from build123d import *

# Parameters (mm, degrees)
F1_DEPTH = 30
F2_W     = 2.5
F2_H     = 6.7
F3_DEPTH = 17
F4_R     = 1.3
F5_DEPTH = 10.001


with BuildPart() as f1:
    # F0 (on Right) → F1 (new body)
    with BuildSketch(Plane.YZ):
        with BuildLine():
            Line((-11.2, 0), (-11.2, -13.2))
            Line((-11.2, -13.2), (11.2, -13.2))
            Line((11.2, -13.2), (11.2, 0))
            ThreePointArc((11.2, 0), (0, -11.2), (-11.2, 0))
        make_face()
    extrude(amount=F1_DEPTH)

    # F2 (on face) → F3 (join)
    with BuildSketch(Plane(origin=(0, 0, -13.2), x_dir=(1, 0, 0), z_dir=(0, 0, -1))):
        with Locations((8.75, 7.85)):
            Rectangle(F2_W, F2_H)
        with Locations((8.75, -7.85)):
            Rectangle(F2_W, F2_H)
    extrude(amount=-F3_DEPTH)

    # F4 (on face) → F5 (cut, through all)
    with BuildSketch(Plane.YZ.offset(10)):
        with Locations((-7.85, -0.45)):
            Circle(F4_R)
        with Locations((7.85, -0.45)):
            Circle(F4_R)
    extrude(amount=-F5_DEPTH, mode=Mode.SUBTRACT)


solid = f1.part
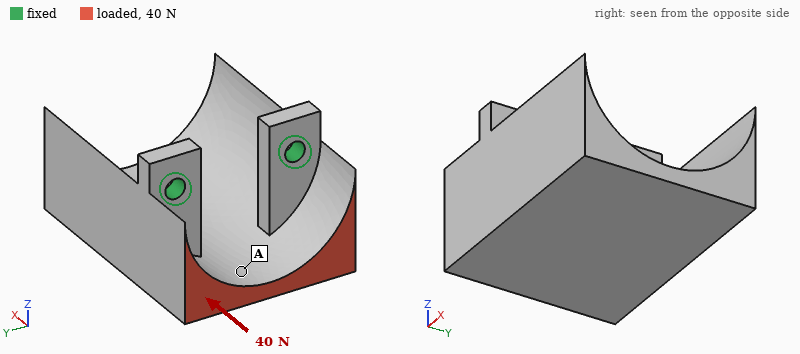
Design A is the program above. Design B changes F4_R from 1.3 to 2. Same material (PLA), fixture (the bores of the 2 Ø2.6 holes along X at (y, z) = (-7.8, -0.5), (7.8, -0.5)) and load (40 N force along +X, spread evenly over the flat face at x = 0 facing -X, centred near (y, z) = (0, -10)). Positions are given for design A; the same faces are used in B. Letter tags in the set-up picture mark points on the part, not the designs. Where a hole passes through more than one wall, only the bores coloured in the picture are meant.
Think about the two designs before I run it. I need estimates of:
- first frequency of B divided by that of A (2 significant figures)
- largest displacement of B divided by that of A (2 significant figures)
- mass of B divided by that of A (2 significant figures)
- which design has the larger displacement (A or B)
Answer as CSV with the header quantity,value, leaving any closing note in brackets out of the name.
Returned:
quantity,value
first frequency of B divided by that of A,1.2
largest displacement of B divided by that of A,0.72
mass of B divided by that of A,0.99
which design has the larger displacement,A
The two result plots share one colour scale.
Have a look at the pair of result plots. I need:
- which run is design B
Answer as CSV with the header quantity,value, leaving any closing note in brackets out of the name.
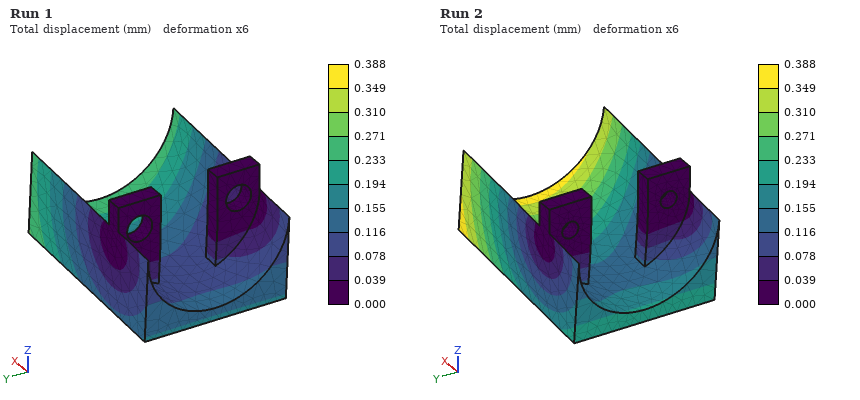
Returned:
quantity,value
which run is design B,Run 1
